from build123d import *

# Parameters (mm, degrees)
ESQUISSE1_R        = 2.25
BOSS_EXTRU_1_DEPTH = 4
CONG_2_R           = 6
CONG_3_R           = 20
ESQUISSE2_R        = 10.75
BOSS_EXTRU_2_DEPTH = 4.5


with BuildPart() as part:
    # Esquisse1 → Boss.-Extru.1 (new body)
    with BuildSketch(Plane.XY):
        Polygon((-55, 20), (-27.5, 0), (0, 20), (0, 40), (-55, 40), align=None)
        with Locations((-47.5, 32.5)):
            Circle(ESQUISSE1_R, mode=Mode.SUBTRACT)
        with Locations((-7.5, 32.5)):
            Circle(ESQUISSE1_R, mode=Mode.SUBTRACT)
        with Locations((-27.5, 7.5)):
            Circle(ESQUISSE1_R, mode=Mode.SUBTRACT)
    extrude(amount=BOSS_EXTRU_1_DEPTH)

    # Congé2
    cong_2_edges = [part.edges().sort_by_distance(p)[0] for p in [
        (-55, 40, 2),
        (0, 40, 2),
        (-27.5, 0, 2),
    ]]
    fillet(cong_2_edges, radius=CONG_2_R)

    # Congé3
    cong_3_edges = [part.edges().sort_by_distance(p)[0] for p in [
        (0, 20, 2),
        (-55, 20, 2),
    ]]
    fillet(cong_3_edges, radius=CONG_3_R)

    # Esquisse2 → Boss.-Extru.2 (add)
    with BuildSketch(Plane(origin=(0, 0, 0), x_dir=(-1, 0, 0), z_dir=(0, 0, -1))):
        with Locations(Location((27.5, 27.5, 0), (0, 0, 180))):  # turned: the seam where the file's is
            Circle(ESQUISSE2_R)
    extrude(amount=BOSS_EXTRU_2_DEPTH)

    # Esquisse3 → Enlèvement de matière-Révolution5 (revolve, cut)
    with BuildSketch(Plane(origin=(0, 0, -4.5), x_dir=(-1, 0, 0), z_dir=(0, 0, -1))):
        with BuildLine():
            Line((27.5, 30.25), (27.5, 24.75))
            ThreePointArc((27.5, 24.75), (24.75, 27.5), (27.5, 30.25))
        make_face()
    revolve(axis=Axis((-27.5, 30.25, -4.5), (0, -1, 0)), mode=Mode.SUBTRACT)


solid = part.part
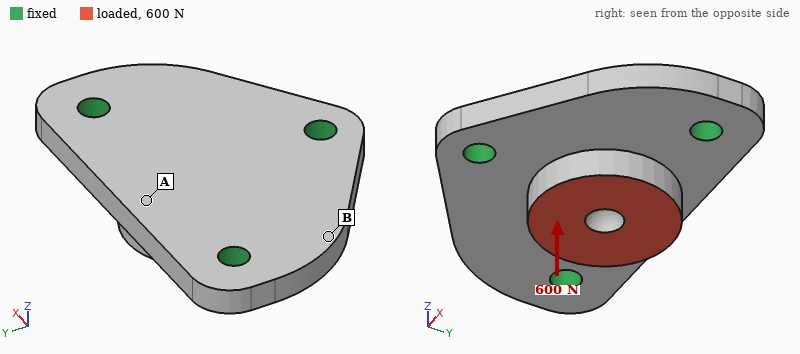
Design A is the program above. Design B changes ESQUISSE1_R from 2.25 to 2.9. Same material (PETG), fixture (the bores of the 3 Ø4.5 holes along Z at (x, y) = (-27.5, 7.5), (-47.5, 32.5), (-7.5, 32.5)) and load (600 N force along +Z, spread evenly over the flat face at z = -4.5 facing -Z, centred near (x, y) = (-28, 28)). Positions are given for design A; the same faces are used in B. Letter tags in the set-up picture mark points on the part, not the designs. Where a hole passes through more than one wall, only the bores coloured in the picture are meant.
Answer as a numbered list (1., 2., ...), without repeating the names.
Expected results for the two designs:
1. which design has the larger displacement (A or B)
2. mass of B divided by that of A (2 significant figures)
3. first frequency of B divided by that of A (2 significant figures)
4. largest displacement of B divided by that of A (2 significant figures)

1. A
2. 0.98
3. 1.1
4. 0.85
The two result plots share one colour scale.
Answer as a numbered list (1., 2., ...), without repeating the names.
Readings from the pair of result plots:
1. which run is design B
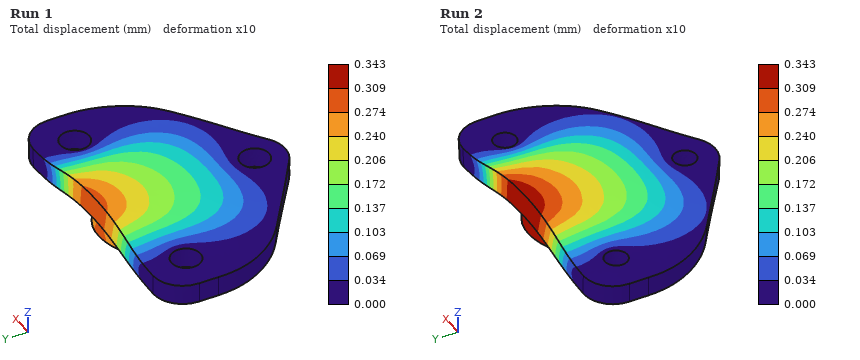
1. Run 1
